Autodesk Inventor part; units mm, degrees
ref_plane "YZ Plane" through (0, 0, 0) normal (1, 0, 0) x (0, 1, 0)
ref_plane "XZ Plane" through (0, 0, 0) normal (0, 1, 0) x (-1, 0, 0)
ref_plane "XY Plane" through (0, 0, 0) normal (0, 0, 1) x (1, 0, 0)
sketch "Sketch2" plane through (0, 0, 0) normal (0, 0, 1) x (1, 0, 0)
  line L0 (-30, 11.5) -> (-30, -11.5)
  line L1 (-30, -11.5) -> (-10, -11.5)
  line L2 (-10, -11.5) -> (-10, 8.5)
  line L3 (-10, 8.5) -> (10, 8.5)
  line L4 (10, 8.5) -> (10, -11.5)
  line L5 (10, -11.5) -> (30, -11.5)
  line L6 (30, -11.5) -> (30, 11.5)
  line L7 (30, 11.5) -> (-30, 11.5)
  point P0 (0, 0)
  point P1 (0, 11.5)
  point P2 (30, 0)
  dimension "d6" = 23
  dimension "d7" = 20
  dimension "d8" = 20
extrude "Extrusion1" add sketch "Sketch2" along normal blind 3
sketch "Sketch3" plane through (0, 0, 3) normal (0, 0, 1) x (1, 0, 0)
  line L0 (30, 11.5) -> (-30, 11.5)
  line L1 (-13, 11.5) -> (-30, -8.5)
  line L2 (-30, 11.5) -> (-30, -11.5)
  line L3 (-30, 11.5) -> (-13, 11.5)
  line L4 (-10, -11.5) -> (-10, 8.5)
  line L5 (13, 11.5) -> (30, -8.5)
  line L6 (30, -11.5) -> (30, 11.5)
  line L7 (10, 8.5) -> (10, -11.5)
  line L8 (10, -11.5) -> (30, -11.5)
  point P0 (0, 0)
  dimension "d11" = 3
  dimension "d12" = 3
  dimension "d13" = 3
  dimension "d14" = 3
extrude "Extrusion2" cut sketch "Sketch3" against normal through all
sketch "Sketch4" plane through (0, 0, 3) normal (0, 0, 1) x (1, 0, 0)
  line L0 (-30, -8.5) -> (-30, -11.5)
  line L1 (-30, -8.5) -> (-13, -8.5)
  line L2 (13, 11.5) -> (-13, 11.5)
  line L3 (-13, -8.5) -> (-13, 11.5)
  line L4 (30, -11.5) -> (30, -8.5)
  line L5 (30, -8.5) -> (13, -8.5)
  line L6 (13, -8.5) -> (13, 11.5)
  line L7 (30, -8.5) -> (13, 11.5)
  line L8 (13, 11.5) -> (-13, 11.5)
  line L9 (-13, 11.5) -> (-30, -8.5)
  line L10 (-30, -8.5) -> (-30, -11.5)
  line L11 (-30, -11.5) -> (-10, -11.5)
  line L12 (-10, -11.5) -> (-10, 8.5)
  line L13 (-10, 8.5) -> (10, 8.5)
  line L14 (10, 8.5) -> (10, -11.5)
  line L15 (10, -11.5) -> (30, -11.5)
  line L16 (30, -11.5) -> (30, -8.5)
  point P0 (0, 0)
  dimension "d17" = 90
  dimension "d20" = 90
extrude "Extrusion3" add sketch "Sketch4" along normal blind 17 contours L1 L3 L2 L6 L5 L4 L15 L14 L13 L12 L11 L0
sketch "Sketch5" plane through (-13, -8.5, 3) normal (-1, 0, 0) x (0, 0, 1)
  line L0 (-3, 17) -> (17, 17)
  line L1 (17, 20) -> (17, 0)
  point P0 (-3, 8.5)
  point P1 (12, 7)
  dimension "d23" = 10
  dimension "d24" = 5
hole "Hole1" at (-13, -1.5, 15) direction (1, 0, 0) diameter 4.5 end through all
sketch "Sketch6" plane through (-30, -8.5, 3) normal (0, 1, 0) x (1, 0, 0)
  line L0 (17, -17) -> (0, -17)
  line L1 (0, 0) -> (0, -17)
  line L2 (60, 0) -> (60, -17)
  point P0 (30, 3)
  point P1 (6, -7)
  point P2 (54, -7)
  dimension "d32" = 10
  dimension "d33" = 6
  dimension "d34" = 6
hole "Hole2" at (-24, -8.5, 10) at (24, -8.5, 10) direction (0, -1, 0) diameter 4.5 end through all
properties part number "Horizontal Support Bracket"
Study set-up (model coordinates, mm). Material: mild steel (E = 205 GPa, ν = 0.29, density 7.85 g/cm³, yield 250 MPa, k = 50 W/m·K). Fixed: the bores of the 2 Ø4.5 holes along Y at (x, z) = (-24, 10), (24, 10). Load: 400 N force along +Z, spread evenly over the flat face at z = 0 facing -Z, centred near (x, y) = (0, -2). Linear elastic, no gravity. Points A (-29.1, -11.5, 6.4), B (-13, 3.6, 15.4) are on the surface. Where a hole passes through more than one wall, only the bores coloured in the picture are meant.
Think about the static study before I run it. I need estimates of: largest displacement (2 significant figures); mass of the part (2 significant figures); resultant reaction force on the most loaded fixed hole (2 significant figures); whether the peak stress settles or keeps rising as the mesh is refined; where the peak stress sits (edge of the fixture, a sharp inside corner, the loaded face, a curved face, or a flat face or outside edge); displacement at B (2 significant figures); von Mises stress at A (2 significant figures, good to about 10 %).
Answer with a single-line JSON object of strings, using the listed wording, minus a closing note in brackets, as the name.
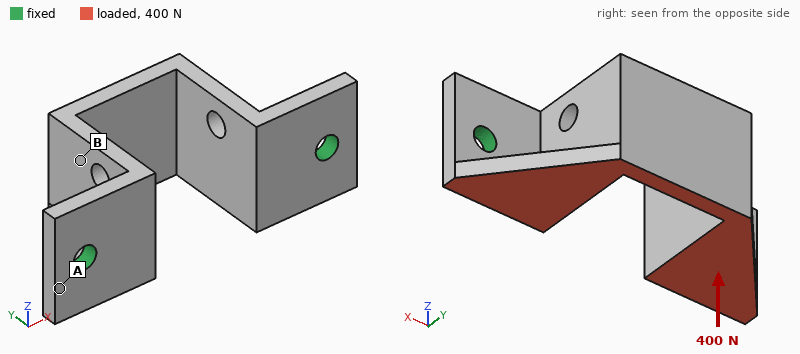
{"largest displacement": "21 µm", "mass of the part": "54 g", "resultant reaction force on the most loaded fixed hole": "200 N", "whether the peak stress settles or keeps rising as the mesh is refined": "keeps rising", "where the peak stress sits": "edge of the fixture", "displacement at B": "14 µm", "von Mises stress at A": "33 MPa"}
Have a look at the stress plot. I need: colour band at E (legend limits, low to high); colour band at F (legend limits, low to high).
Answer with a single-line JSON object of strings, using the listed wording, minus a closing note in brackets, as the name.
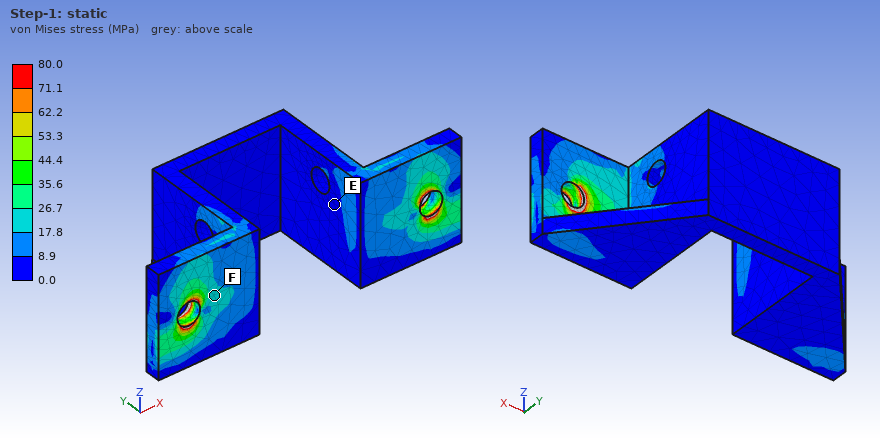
{"colour band at E": "0.0 to 8.9 MPa", "colour band at F": "17.8 to 26.7 MPa"}
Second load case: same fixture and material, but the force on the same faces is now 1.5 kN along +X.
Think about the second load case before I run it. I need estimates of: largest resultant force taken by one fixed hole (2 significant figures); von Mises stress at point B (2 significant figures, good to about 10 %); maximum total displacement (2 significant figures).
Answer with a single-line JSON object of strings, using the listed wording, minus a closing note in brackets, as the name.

{"largest resultant force taken by one fixed hole": "780 N", "von Mises stress at point B": "20 MPa", "maximum total displacement": "31 µm"}
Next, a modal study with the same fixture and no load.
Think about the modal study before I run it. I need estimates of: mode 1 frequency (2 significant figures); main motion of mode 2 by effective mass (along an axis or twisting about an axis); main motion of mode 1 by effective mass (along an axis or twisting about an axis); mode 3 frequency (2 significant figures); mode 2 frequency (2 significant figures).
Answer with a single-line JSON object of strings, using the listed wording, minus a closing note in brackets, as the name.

{"mode 1 frequency": "3300 Hz", "main motion of mode 2 by effective mass": "along X", "main motion of mode 1 by effective mass": "along Z", "mode 3 frequency": "6900 Hz", "mode 2 frequency": "5600 Hz"}
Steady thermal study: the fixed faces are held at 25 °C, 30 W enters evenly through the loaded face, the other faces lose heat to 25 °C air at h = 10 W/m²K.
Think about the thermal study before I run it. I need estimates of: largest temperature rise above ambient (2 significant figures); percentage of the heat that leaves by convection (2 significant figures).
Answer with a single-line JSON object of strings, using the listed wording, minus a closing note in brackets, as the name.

{"largest temperature rise above ambient": "68 K", "percentage of the heat that leaves by convection": "6.5 %"}
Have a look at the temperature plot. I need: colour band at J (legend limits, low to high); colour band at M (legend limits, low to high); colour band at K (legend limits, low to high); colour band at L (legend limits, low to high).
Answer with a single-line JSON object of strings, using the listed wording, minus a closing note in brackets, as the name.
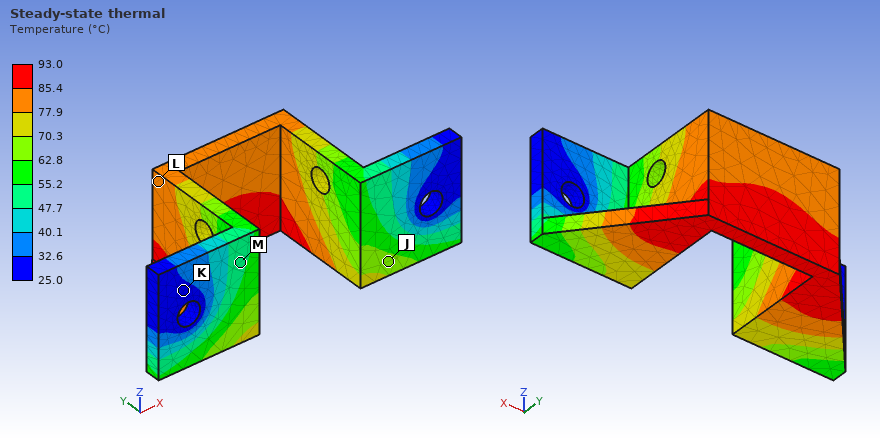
{"colour band at J": "62.8 to 70.3 °C", "colour band at M": "47.7 to 55.2 °C", "colour band at K": "25.0 to 32.6 °C", "colour band at L": "77.9 to 85.4 °C"}
